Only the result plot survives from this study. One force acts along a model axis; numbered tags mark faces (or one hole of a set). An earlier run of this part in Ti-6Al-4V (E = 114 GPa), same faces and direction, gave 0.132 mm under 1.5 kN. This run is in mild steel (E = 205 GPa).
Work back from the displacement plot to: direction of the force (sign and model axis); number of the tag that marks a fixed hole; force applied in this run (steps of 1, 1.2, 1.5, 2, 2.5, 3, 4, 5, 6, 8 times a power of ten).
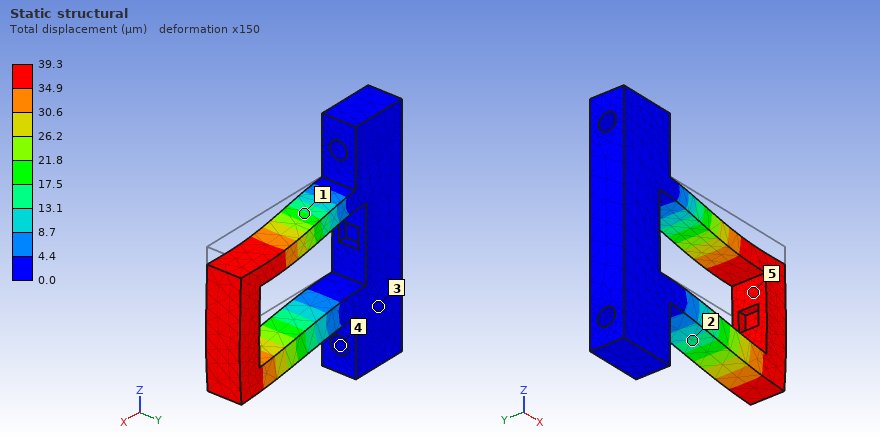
-Z
4
800 N
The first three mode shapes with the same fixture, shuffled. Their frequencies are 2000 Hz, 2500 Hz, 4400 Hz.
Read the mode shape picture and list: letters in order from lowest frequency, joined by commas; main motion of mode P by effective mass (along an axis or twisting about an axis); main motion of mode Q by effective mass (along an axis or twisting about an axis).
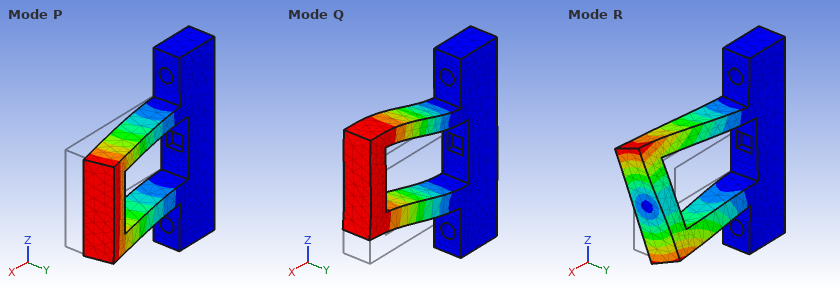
P, Q, R
along Y
along Z
